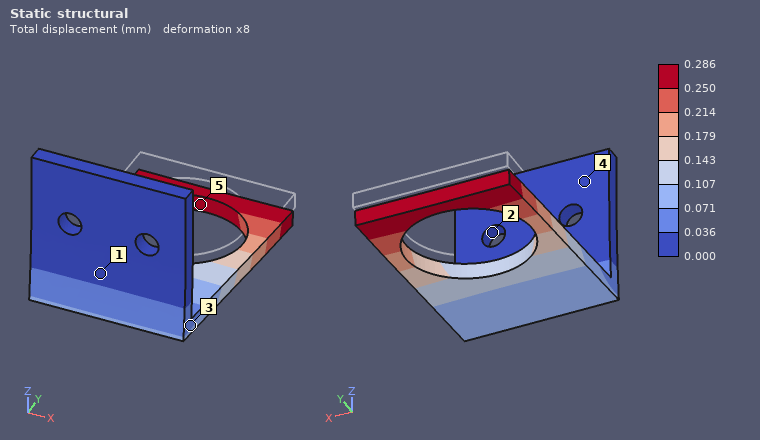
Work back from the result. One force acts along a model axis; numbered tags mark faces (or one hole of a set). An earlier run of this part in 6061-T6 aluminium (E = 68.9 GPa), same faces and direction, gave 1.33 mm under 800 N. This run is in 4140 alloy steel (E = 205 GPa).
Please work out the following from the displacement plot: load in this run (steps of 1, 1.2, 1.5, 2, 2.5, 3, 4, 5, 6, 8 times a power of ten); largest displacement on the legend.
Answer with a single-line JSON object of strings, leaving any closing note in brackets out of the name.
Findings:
{"load in this run": "500 N", "largest displacement on the legend": "0.286 mm"}
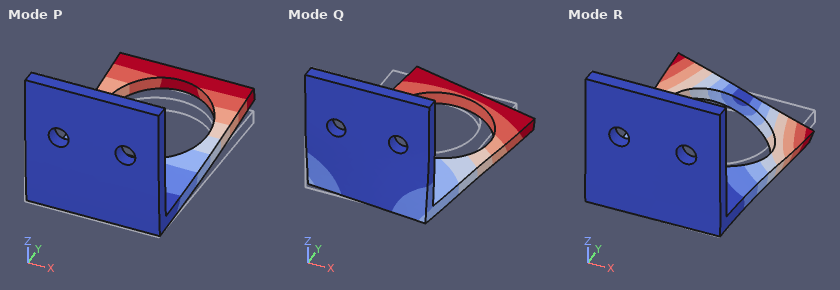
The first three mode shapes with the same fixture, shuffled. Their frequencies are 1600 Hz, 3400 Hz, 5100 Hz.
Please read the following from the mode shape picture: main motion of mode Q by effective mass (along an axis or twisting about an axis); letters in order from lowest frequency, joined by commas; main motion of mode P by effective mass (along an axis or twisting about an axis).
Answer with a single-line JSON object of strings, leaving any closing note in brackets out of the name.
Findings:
{"main motion of mode Q by effective mass": "along X", "letters in order from lowest frequency, joined by commas": "P, Q, R", "main motion of mode P by effective mass": "along Z"}
